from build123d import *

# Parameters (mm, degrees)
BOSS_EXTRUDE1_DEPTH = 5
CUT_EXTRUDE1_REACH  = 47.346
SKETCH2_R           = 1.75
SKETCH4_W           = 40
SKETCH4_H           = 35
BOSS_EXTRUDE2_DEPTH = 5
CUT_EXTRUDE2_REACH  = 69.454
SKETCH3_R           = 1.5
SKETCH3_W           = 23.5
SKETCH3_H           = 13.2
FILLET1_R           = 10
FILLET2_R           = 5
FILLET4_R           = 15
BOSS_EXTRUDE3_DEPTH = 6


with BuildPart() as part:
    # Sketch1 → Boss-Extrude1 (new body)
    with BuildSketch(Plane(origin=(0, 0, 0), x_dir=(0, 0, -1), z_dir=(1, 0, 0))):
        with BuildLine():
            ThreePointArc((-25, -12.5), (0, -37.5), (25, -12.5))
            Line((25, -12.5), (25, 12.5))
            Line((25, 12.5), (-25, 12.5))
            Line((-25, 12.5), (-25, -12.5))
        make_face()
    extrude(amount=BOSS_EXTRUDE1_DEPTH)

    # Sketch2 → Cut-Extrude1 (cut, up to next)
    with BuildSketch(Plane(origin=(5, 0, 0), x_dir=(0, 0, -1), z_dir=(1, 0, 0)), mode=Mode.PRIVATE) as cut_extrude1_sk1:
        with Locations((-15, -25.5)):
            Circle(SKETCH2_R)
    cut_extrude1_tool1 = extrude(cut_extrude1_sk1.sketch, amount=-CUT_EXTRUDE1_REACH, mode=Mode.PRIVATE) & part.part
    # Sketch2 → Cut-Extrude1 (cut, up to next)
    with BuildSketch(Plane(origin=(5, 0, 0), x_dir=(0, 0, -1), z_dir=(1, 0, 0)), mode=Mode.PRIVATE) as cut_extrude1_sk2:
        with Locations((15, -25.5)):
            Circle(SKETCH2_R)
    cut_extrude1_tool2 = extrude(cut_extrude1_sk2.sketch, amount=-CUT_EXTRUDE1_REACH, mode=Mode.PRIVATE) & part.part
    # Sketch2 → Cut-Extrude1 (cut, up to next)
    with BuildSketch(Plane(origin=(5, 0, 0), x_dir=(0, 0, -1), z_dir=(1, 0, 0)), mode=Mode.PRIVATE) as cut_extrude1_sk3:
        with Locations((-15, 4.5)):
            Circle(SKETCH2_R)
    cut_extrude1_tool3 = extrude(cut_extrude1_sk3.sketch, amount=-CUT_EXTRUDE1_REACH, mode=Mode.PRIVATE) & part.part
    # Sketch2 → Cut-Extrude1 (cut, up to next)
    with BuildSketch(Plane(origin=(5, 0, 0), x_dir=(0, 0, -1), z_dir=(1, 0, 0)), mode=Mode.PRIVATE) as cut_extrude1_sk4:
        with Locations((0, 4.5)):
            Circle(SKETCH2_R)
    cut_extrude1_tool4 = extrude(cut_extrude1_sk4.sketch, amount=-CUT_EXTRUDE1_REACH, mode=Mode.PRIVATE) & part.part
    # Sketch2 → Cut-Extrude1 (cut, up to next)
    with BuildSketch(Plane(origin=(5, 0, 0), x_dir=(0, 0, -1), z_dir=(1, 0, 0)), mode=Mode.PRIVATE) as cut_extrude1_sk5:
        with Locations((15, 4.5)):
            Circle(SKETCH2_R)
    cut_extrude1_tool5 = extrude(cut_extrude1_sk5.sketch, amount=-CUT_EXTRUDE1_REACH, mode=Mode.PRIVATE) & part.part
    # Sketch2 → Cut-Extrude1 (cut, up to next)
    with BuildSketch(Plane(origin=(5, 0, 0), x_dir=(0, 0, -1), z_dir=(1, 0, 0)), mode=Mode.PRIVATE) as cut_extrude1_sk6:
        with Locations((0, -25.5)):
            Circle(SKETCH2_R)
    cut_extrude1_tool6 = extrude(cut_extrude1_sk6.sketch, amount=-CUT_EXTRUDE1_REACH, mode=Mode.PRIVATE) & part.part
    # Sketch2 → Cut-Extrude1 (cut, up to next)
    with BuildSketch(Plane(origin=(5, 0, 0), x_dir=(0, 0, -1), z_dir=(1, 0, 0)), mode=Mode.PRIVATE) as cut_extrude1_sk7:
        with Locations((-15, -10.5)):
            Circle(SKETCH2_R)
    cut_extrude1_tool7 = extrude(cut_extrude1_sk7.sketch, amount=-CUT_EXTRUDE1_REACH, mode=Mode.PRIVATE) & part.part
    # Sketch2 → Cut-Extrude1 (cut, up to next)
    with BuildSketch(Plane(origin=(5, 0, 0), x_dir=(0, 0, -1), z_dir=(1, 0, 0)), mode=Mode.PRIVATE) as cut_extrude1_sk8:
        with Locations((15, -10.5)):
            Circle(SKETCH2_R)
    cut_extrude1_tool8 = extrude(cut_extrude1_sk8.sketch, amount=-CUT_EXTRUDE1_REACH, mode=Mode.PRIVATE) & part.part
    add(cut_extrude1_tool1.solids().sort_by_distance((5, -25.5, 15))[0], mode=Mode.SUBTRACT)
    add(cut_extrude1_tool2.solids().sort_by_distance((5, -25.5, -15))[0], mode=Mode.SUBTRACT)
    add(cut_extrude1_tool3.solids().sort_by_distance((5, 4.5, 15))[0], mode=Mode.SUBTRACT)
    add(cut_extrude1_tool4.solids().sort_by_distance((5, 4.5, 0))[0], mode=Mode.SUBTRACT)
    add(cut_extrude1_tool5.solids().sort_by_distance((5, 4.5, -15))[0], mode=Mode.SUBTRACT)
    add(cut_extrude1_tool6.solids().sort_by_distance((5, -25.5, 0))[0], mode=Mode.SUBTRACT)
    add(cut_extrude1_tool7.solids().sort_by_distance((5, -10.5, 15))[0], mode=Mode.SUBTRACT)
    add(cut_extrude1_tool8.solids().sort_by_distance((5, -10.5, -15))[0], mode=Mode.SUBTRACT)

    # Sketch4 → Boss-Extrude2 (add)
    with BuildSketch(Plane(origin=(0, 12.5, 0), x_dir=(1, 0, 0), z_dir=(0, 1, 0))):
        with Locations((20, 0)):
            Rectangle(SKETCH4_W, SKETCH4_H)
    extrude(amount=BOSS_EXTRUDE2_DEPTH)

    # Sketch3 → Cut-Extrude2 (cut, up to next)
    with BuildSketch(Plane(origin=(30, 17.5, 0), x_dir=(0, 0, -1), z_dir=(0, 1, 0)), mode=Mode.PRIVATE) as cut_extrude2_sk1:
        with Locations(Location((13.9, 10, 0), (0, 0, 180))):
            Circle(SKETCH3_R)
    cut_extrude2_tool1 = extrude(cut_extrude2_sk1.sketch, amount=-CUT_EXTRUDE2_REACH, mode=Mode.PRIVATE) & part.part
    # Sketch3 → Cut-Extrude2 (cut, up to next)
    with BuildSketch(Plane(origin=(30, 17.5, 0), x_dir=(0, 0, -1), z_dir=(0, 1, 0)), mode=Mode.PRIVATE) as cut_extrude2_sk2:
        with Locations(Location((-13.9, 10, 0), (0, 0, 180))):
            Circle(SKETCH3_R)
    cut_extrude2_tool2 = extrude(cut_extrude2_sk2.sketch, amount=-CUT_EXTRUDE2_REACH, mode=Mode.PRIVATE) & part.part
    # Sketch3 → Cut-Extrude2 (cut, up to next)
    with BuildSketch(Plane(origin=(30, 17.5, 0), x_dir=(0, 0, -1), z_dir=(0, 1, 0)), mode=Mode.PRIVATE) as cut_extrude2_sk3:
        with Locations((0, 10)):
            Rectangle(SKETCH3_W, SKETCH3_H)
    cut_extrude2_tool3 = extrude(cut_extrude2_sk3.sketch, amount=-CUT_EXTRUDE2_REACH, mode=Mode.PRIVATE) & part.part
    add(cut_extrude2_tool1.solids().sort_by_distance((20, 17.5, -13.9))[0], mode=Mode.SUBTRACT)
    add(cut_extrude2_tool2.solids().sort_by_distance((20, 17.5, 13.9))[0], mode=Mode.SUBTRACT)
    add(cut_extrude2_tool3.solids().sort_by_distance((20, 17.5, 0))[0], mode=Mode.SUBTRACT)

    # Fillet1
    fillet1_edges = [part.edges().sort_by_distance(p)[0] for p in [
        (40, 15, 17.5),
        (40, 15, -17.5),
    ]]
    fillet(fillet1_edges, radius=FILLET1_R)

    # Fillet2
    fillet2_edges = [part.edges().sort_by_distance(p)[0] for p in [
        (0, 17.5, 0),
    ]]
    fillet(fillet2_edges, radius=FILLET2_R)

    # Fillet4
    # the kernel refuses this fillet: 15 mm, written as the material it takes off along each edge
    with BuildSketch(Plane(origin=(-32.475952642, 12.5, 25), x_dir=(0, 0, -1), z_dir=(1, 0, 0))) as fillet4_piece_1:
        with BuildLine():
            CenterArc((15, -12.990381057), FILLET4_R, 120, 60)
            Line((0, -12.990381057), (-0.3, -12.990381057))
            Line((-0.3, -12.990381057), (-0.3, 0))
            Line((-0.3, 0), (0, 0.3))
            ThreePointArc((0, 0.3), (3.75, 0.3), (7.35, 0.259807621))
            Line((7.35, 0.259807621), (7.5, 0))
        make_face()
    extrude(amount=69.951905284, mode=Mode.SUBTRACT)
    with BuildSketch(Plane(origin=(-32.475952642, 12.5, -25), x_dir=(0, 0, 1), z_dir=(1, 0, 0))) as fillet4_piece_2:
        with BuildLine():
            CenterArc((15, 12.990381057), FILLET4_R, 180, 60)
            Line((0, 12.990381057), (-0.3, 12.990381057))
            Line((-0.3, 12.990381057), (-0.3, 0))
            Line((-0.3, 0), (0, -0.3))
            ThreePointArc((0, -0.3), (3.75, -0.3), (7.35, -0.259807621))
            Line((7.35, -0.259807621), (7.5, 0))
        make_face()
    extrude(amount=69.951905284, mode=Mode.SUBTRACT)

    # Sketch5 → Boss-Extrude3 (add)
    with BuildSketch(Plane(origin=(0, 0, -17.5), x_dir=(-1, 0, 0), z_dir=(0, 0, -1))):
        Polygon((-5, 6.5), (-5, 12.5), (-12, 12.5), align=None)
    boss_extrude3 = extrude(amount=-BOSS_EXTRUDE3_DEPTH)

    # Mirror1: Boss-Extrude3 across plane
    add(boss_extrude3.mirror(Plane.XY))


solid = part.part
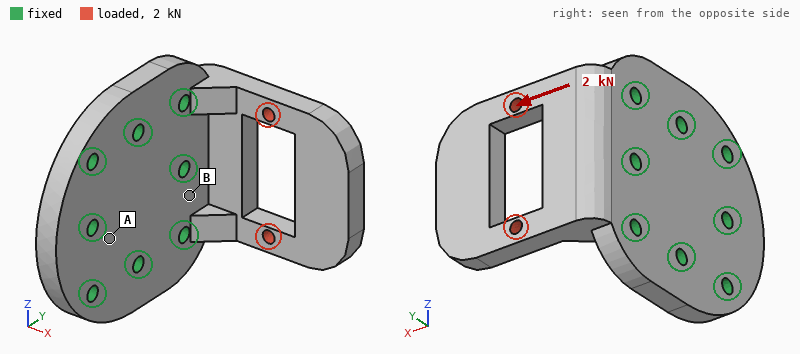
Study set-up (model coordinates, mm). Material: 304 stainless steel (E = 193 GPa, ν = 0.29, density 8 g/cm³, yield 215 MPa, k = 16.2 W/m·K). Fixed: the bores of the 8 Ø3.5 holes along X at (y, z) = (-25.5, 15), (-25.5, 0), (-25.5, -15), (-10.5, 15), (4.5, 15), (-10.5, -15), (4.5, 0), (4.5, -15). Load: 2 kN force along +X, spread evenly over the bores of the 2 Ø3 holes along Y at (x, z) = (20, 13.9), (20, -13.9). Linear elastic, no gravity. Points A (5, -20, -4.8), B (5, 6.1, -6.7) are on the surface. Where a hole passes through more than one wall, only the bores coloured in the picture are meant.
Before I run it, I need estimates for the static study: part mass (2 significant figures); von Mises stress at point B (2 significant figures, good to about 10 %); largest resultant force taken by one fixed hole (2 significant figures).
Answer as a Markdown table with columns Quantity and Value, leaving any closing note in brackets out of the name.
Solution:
| Quantity | Value |
|---|---|
| part mass | 130 g |
| von Mises stress at point B | 46 MPa |
| largest resultant force taken by one fixed hole | 820 N |
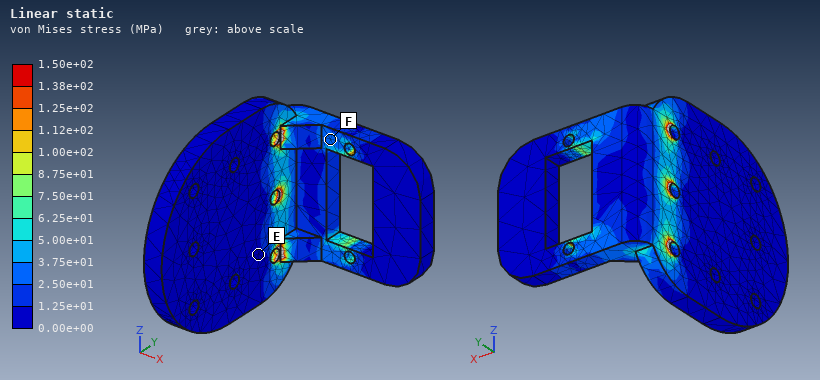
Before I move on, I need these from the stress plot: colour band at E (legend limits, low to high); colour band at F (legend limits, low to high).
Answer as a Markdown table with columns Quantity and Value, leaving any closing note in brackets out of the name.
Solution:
| Quantity | Value |
|---|---|
| colour band at E | 0.00e+00 to 1.25e+01 MPa |
| colour band at F | 2.50e+01 to 3.75e+01 MPa |
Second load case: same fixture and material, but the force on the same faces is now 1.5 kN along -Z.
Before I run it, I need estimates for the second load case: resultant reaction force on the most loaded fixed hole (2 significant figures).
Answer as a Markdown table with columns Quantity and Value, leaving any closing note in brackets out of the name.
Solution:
| Quantity | Value |
|---|---|
| resultant reaction force on the most loaded fixed hole | 1.0 kN |
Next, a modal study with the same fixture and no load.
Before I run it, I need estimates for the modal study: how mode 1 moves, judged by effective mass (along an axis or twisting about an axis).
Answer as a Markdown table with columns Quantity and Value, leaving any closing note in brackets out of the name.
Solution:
| Quantity | Value |
|---|---|
| how mode 1 moves, judged by effective mass | along Y |
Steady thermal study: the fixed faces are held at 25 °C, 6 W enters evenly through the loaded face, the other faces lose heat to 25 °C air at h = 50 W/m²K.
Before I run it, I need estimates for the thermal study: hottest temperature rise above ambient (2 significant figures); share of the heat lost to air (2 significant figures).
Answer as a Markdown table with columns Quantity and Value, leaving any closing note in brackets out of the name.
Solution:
| Quantity | Value |
|---|---|
| hottest temperature rise above ambient | 51 K |
| share of the heat lost to air | 57 % |
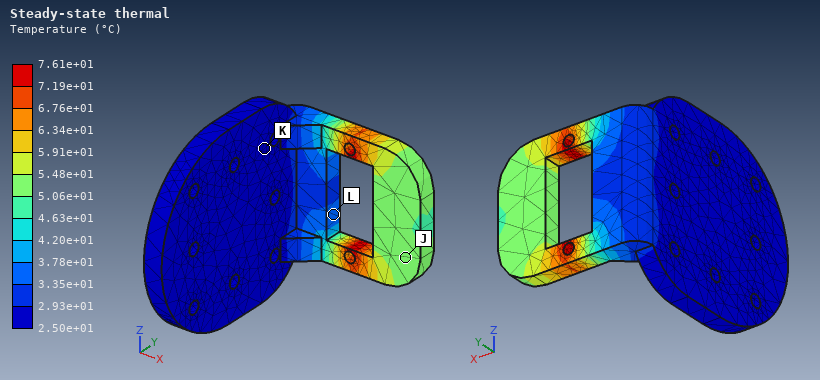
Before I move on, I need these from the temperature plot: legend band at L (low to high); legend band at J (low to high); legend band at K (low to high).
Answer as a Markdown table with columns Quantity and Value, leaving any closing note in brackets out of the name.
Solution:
| Quantity | Value |
|---|---|
| legend band at L | 3.35e+01 to 3.78e+01 °C |
| legend band at J | 5.06e+01 to 5.48e+01 °C |
| legend band at K | 2.50e+01 to 2.93e+01 °C |
